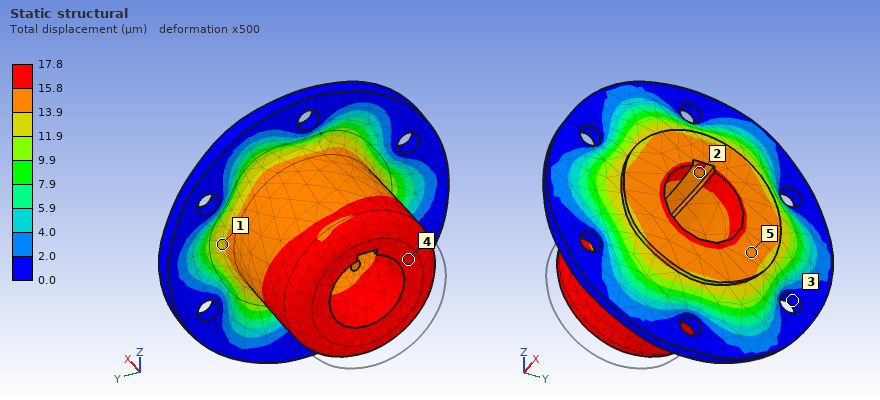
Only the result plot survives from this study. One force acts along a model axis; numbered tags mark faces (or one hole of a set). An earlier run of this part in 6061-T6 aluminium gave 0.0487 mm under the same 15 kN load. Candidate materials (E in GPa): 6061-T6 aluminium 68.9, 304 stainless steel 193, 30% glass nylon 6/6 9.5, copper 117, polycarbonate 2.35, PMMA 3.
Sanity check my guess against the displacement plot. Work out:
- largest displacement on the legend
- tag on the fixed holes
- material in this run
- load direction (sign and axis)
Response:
17.8 µm
3
304 stainless steel
+X
